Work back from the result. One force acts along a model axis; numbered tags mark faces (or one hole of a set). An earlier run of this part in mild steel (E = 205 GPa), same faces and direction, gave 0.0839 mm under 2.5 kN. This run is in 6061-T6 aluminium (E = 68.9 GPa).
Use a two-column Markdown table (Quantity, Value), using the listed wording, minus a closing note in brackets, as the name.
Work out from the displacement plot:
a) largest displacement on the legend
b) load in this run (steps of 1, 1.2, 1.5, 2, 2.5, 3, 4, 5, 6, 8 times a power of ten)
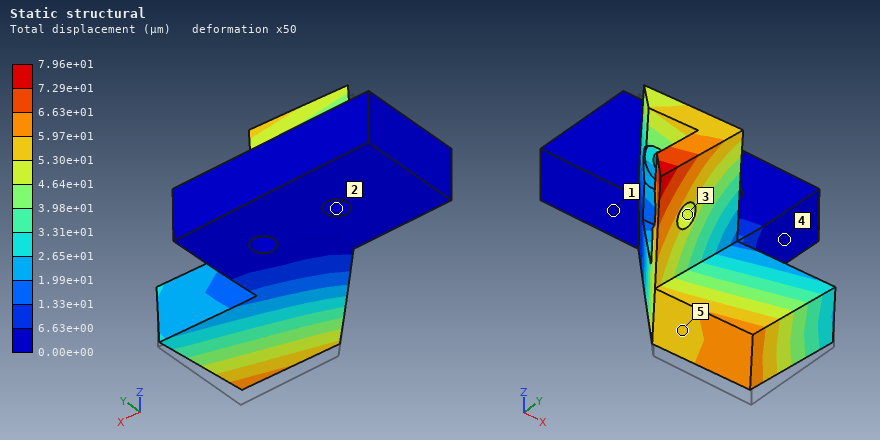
| Quantity | Value |
|---|---|
| largest displacement on the legend | 7.96e+01 µm |
| load in this run | 800 N |
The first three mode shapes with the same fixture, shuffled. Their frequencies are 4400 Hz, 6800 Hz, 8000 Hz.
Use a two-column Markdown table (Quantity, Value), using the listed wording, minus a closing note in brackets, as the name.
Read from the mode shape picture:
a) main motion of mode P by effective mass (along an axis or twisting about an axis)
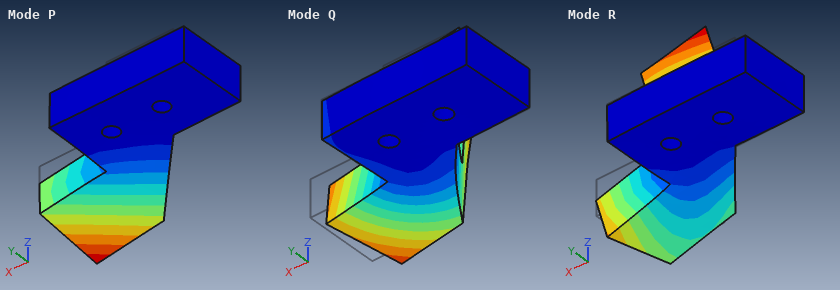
| Quantity | Value |
|---|---|
| main motion of mode P by effective mass | along Z |
